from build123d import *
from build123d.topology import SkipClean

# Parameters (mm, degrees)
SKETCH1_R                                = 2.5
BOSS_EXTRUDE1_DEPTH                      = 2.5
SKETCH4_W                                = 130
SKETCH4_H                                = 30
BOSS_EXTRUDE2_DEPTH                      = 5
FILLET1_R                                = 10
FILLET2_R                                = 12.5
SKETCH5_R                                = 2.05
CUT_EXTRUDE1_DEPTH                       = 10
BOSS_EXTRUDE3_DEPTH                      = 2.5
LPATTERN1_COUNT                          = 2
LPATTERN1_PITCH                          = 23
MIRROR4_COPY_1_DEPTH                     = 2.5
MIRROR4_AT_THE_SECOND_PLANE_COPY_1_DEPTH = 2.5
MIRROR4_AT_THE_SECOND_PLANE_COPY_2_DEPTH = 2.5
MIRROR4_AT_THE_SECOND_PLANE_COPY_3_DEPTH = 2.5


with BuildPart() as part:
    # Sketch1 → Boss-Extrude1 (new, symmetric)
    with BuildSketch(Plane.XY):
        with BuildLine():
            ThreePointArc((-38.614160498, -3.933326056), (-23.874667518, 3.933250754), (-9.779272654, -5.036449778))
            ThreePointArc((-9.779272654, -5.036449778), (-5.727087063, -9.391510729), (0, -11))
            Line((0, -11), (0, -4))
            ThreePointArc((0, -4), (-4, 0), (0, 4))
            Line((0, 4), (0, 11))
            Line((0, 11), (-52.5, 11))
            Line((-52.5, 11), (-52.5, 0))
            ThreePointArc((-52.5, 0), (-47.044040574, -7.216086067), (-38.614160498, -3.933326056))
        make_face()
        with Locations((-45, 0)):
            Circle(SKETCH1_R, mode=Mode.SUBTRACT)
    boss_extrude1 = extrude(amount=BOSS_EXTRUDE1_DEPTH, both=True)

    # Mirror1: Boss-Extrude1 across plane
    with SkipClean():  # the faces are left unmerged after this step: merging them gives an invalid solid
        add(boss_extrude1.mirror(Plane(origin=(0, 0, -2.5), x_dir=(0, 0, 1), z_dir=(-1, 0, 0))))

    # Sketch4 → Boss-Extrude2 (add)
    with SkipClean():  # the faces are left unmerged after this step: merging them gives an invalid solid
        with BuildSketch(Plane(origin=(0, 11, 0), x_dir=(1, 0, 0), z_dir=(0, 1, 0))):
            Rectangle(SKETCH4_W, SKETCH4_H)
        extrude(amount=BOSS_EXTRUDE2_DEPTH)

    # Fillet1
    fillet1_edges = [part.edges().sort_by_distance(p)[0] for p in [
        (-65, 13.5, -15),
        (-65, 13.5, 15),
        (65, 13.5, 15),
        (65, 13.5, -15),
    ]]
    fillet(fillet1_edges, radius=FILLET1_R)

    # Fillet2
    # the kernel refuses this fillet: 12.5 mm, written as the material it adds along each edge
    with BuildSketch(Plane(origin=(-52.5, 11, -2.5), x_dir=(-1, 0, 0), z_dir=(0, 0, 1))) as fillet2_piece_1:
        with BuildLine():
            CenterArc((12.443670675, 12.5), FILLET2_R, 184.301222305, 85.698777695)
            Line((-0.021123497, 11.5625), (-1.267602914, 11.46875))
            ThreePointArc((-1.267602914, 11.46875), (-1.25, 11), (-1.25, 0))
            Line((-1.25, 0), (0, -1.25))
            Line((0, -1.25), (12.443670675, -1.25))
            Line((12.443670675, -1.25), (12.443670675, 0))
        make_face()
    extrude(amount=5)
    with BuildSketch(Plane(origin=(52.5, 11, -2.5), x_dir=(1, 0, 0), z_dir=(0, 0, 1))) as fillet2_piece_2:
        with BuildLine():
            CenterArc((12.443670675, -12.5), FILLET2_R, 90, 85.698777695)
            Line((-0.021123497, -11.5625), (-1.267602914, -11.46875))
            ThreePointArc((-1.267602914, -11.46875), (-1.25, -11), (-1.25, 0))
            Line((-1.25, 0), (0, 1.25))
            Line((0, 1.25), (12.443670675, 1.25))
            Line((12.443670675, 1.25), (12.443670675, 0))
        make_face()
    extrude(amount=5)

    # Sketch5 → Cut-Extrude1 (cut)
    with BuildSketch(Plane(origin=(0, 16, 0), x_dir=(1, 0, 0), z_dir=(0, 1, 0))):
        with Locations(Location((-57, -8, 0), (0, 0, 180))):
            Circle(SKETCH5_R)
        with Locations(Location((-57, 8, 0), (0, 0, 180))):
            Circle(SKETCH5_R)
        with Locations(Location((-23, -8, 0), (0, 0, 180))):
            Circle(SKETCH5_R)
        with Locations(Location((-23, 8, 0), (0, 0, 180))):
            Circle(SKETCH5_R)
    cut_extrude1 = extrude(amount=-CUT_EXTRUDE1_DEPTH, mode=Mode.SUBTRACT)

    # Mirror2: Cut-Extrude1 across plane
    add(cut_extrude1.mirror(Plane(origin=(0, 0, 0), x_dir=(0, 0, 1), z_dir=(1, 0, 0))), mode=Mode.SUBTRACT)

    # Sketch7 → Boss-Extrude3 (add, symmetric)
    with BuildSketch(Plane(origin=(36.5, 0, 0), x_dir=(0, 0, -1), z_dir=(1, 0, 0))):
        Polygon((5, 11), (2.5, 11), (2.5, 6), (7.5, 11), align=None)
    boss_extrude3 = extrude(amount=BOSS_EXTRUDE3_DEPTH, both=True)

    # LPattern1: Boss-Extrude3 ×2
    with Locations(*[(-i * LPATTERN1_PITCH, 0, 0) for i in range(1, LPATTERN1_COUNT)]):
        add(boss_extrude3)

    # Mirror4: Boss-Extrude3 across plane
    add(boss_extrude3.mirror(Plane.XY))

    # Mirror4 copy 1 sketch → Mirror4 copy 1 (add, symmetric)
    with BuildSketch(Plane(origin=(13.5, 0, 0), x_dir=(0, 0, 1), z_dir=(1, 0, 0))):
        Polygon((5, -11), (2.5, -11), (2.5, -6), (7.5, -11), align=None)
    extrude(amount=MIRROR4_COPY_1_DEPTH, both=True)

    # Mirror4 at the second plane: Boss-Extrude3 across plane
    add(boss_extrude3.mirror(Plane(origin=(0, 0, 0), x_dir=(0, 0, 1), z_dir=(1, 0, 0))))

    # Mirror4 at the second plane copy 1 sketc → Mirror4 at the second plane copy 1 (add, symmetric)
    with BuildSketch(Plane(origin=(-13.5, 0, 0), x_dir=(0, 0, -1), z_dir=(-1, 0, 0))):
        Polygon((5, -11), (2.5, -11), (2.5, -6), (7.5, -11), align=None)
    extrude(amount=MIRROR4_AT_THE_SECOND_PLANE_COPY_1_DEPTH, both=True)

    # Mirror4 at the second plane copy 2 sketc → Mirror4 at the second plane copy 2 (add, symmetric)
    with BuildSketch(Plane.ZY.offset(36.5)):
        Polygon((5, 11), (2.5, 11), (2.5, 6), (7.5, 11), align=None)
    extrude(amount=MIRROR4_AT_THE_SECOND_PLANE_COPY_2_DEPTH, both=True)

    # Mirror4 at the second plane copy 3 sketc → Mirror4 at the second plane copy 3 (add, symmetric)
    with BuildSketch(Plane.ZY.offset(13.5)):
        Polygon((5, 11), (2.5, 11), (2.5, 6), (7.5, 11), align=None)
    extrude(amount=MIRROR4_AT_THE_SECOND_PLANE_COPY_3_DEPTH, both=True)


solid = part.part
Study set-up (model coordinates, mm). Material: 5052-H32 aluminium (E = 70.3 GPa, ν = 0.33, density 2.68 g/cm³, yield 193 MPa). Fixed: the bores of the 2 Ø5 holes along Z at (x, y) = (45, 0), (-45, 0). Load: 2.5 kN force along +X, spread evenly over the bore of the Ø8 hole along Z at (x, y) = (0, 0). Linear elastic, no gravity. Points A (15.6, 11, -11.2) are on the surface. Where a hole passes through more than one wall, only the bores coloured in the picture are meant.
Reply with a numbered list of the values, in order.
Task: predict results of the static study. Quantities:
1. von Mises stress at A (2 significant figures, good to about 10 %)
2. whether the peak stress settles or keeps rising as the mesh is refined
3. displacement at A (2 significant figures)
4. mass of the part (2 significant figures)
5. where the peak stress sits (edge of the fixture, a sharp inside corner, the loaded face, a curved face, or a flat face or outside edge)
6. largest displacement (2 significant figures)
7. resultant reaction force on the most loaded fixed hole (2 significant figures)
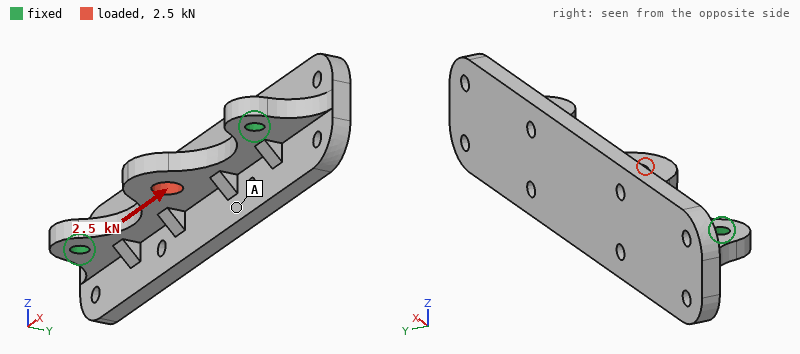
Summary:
1. 11 MPa
2. keeps rising
3. 23 µm
4. 70 g
5. edge of the fixture
6. 44 µm
7. 1.3 kN
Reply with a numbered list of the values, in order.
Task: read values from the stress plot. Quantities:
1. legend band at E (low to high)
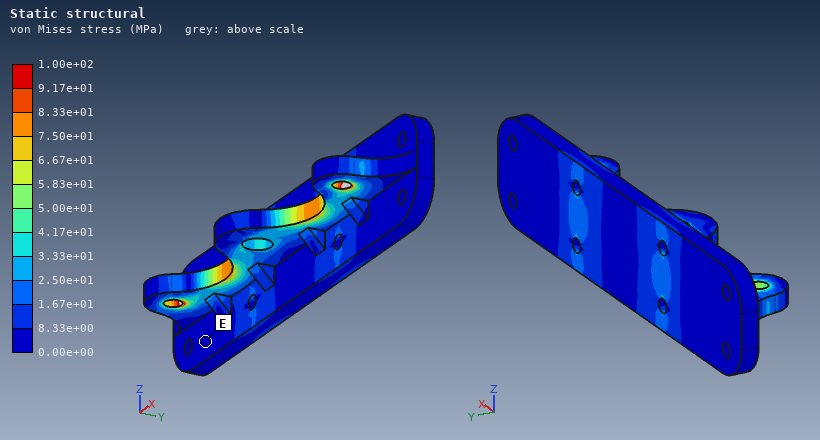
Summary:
1. 0.00e+00 to 8.33e+00 MPa
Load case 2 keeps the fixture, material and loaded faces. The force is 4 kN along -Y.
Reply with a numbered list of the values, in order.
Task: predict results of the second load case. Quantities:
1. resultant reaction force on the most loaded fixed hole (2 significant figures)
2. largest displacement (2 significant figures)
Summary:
1. 3.3 kN
2. 100 µm
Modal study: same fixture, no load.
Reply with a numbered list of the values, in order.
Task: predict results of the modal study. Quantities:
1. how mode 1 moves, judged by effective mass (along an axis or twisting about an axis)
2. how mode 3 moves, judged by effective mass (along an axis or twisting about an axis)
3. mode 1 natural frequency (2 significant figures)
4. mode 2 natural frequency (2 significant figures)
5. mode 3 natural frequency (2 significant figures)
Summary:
1. along Z
2. along Z
3. 3000 Hz
4. 5100 Hz
5. 5300 Hz
